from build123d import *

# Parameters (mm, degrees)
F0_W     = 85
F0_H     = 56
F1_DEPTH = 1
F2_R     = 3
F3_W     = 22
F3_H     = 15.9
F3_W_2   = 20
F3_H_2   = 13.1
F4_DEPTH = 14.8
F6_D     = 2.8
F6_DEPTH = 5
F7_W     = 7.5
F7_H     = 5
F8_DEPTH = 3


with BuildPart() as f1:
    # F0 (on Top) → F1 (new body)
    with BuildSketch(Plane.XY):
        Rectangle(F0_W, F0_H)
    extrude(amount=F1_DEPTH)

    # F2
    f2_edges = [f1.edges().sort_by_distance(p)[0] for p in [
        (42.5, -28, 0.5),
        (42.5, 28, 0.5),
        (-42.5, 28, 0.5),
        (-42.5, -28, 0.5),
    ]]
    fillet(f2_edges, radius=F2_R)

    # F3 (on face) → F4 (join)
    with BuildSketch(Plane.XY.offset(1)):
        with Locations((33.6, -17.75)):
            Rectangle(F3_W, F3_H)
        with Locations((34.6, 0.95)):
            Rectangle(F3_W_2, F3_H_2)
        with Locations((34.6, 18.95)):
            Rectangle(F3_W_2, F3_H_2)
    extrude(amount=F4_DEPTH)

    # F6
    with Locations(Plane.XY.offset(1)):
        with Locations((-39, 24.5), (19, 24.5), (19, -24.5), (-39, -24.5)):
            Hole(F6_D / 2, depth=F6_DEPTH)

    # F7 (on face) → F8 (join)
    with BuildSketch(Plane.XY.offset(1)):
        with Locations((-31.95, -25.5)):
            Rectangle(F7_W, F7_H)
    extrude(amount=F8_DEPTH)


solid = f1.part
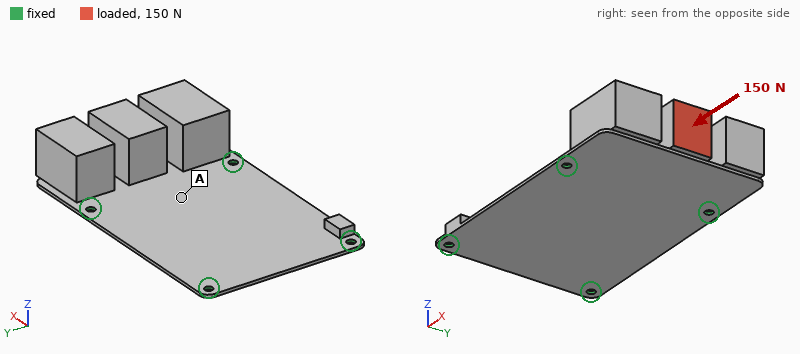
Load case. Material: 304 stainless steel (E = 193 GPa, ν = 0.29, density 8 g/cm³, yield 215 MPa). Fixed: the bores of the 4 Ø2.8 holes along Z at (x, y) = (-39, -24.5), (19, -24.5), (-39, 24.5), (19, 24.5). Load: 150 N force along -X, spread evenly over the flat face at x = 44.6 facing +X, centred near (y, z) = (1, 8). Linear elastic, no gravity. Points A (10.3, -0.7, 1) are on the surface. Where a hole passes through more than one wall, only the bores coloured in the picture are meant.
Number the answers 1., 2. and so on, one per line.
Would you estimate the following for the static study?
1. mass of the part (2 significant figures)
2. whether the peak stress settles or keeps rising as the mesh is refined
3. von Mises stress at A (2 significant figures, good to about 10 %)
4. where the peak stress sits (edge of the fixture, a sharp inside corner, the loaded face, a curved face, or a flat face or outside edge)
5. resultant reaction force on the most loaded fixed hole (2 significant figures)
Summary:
1. 140 g
2. keeps rising
3. 31 MPa
4. edge of the fixture
5. 63 N
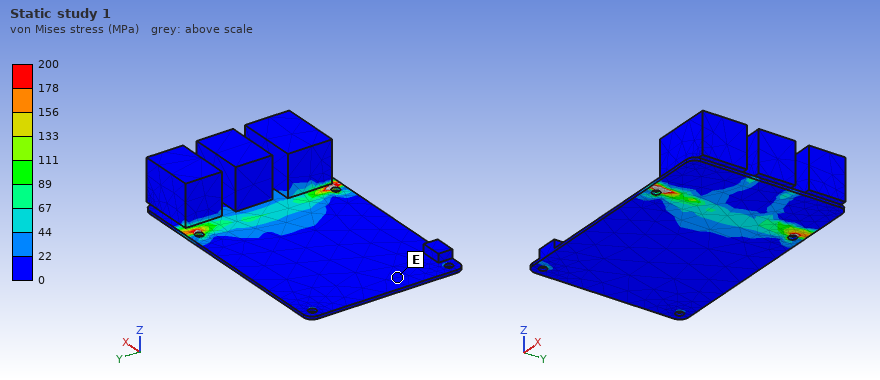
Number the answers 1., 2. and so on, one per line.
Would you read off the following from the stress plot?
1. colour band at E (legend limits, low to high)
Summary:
1. 0 to 22 MPa
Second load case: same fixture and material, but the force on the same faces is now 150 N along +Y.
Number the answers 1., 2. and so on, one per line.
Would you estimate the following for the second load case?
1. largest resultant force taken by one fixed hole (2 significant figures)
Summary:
1. 110 N
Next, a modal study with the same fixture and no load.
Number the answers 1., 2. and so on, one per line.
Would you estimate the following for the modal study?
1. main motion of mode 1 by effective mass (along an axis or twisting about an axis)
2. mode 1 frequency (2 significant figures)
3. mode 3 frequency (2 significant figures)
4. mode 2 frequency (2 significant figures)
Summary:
1. along Z
2. 300 Hz
3. 1300 Hz
4. 980 Hz
